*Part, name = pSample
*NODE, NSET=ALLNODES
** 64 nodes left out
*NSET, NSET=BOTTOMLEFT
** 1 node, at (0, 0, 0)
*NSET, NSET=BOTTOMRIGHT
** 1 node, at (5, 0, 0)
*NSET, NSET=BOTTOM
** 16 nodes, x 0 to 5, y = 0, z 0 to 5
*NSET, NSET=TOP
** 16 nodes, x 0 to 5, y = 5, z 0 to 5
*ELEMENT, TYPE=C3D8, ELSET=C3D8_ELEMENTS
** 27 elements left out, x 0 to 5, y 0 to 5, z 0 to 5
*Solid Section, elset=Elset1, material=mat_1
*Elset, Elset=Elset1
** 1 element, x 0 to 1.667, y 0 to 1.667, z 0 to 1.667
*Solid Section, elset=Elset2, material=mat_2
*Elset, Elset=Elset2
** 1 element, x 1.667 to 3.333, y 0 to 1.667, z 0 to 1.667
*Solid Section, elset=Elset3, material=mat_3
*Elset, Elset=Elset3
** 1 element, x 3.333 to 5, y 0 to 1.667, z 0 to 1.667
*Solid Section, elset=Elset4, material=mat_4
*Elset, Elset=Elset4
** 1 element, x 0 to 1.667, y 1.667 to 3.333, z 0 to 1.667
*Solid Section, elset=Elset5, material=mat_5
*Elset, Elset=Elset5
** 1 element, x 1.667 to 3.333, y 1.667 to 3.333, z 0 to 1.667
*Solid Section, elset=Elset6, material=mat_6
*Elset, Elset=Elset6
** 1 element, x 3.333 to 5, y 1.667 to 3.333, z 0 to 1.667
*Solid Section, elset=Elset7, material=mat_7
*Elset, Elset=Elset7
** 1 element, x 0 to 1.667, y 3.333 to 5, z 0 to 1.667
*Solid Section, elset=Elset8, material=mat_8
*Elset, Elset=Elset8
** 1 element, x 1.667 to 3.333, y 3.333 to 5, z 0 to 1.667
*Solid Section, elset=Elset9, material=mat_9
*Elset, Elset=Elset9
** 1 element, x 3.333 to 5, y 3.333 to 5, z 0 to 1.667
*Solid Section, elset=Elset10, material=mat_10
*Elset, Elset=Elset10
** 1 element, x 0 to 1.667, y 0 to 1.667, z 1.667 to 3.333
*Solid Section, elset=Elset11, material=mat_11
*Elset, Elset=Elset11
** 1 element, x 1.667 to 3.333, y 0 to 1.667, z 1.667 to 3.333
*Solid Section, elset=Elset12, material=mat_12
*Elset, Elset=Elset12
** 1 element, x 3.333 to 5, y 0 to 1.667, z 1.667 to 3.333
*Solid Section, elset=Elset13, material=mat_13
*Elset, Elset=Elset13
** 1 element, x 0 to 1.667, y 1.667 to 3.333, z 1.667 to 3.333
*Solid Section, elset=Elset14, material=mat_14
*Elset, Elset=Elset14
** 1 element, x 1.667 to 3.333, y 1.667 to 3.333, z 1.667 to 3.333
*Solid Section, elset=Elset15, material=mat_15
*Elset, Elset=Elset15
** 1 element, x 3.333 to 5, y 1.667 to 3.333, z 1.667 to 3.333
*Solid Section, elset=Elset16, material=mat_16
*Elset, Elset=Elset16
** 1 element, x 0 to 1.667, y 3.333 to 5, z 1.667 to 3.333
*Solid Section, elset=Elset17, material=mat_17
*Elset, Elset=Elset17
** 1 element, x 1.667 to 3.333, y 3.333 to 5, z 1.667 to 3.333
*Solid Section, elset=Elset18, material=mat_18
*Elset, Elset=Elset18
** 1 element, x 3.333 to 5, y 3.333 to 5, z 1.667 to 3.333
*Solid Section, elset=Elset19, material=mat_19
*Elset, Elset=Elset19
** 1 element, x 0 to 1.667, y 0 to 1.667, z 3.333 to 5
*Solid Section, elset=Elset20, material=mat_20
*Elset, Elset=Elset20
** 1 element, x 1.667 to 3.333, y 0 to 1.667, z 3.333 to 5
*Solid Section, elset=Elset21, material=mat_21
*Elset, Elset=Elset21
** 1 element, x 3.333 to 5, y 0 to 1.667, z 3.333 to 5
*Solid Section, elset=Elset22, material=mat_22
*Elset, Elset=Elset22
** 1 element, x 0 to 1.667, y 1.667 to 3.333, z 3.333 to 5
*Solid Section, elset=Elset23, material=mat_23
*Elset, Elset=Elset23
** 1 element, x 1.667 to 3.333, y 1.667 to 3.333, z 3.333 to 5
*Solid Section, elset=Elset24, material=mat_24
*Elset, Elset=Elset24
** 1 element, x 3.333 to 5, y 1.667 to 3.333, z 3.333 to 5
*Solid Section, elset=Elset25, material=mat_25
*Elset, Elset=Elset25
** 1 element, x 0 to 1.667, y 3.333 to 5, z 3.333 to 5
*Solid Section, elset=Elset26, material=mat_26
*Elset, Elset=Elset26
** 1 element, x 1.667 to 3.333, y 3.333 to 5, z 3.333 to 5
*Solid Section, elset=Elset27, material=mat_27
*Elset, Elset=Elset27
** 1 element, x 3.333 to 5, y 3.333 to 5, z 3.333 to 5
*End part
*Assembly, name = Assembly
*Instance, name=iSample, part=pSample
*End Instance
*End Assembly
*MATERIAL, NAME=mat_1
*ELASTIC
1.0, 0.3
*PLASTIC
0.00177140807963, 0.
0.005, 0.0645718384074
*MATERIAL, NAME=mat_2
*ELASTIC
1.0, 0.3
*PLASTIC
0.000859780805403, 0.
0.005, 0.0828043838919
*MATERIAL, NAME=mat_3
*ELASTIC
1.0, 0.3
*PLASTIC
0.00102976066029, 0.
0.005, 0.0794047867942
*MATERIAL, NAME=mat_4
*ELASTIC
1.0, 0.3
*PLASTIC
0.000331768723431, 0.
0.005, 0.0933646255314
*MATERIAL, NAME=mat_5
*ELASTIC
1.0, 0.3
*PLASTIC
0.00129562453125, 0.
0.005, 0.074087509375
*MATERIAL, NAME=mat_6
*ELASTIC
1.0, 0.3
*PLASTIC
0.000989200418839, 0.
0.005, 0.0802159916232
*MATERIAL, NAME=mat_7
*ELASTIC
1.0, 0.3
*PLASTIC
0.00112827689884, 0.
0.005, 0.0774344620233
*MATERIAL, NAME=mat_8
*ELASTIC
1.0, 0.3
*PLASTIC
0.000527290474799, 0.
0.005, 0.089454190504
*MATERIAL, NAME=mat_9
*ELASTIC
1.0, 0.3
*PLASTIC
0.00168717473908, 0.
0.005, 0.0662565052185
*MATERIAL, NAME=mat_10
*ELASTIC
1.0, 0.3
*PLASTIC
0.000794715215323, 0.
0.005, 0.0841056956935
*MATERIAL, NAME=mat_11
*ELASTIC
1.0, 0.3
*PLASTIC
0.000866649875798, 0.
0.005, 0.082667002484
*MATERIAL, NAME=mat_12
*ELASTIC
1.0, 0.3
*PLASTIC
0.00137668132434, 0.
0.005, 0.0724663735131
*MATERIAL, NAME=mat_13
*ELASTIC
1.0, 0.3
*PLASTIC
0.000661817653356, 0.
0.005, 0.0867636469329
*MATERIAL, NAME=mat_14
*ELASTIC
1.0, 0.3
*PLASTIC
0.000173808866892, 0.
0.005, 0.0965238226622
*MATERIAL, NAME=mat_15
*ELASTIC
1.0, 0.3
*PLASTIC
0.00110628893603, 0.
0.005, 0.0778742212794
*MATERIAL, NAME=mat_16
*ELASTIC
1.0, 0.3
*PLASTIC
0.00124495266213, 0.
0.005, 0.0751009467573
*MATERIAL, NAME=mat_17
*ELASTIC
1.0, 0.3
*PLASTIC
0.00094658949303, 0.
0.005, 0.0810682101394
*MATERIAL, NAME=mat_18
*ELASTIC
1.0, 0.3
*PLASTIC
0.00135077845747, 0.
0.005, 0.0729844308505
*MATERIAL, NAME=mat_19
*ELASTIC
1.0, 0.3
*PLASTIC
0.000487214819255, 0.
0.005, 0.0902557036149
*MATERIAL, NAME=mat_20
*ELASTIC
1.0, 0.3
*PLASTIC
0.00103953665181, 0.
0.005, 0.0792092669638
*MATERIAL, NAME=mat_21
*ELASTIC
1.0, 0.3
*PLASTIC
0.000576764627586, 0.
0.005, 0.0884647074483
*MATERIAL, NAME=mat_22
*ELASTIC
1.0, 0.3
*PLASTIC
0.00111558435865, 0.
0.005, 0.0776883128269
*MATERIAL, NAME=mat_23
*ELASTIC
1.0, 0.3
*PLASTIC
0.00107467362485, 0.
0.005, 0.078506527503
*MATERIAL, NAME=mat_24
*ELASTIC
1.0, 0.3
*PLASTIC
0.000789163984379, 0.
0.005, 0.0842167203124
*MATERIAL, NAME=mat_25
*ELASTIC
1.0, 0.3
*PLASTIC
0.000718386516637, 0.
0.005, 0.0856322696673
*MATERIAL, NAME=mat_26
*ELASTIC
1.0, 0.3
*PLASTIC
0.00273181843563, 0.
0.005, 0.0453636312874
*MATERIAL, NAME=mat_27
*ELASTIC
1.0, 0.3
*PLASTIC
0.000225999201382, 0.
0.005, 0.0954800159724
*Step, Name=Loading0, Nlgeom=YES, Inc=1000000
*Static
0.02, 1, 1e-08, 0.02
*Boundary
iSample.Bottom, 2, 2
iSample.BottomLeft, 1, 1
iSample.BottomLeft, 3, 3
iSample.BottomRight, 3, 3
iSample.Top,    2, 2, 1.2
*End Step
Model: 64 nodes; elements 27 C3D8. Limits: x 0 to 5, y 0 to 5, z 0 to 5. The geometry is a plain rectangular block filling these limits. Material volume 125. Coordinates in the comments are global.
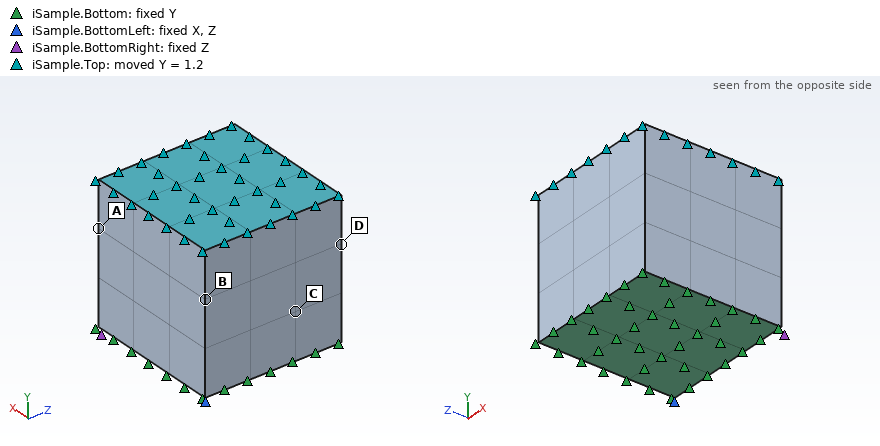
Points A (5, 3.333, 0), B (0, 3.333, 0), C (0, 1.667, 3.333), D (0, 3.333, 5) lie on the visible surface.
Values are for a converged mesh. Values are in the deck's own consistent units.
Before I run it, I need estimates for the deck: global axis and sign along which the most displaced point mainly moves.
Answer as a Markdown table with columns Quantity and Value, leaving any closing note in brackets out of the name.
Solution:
| Quantity | Value |
|---|---|
| global axis and sign along which the most displaced point mainly moves | +Y |
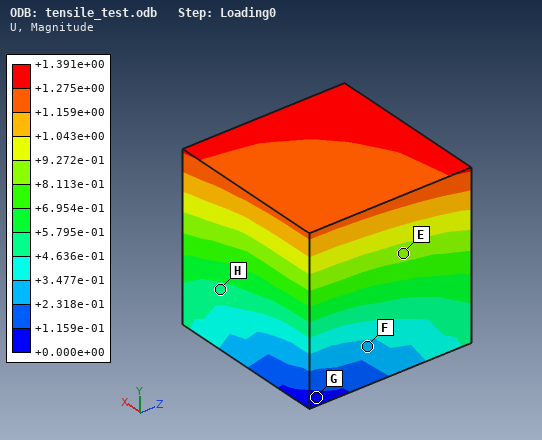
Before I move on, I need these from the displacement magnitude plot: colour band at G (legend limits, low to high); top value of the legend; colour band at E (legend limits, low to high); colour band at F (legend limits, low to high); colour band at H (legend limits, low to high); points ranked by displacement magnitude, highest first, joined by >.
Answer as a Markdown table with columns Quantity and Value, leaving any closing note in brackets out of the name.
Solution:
| Quantity | Value |
|---|---|
| colour band at G | +0.000e+00 to +1.159e-01 |
| top value of the legend | +1.391e+00 |
| colour band at E | +8.113e-01 to +9.272e-01 |
| colour band at F | +2.318e-01 to +3.477e-01 |
| colour band at H | +4.636e-01 to +5.795e-01 |
| points ranked by displacement magnitude, highest first, joined by > | E > H > F > G |
